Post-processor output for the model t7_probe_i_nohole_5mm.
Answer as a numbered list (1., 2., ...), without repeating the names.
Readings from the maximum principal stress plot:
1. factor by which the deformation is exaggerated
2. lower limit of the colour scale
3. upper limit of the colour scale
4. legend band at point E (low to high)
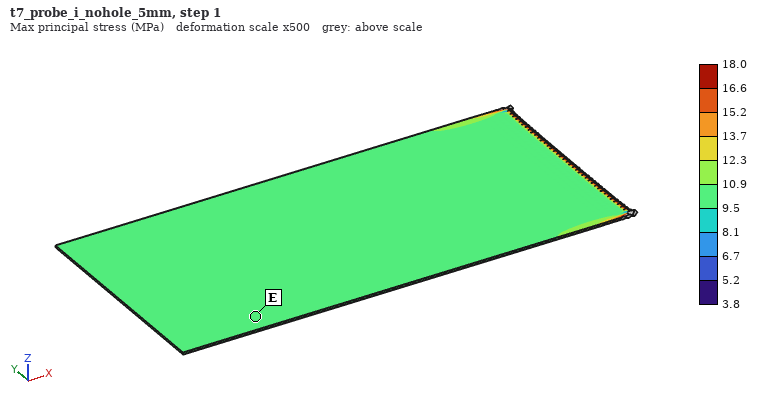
1. 500
2. 3.8 MPa
3. 18.0 MPa
4. 9.5 to 10.9 MPa
